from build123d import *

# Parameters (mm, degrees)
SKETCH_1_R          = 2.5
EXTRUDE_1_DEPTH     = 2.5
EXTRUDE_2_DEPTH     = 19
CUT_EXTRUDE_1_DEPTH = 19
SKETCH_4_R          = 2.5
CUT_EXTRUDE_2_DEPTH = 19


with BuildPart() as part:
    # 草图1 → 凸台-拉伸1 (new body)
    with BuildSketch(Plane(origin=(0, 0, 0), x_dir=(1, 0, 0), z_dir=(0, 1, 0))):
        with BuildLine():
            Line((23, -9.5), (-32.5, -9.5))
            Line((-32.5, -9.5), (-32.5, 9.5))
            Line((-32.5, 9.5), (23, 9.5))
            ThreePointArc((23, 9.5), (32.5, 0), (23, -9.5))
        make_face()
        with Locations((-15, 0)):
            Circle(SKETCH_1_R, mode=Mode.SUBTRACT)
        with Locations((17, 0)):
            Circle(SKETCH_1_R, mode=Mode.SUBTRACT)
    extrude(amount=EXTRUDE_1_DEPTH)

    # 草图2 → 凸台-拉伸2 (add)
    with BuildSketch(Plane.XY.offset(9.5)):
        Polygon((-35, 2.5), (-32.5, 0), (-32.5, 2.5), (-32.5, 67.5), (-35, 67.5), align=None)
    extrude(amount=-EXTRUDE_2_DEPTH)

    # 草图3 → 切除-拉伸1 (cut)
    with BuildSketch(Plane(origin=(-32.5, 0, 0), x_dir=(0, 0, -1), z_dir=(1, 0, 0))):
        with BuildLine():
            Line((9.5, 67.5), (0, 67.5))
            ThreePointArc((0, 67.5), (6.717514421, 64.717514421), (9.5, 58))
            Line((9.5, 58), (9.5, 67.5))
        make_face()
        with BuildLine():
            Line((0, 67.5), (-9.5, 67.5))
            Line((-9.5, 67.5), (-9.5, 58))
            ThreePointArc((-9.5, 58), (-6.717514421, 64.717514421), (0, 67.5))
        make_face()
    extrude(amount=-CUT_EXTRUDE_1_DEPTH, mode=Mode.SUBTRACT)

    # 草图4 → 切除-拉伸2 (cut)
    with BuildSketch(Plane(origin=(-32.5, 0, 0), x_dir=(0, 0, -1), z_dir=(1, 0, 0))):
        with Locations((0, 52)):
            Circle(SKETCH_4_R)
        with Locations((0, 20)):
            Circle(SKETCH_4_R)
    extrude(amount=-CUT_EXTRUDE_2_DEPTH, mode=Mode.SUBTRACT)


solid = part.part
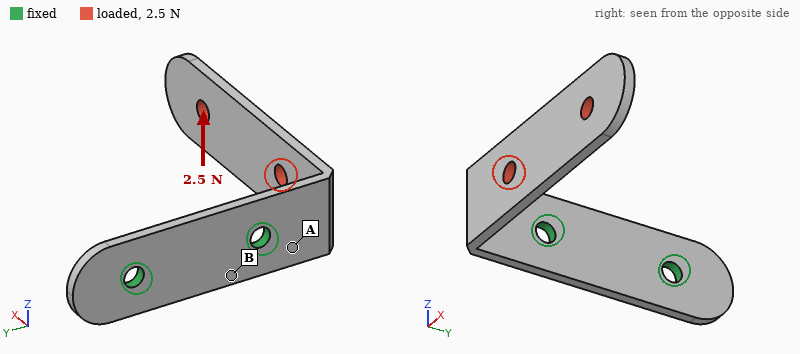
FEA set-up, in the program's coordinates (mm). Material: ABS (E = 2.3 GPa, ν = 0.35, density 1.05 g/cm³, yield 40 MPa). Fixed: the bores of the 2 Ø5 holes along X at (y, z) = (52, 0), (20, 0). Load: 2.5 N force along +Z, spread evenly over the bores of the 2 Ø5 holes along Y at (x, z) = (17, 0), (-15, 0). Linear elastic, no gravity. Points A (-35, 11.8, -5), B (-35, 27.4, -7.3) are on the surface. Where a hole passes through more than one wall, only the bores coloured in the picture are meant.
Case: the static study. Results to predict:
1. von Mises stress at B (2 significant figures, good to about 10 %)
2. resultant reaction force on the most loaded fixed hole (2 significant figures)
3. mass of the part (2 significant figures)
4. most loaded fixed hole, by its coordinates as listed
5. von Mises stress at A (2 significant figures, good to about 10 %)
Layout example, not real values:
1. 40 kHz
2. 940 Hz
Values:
1. 0.63 MPa
2. 3.4 N
3. 6.1 g
4. (20, 0)
5. 3.1 MPa
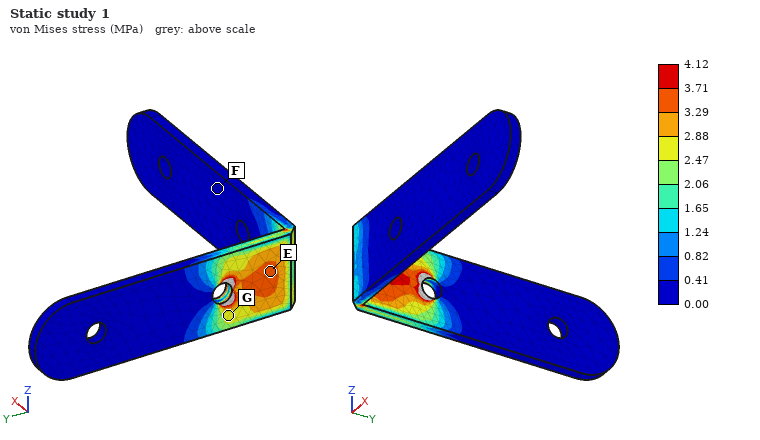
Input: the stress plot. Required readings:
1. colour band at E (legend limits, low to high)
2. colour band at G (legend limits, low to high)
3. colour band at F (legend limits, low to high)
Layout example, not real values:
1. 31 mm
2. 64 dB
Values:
1. 3.29 to 3.71 MPa
2. 2.47 to 2.88 MPa
3. 0.00 to 0.41 MPa
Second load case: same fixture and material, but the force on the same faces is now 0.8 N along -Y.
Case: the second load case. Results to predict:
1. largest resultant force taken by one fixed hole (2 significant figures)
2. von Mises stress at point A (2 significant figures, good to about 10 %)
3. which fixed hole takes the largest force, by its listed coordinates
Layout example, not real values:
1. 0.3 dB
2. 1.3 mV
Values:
1. 0.73 N
2. 1.3 MPa
3. (20, 0)
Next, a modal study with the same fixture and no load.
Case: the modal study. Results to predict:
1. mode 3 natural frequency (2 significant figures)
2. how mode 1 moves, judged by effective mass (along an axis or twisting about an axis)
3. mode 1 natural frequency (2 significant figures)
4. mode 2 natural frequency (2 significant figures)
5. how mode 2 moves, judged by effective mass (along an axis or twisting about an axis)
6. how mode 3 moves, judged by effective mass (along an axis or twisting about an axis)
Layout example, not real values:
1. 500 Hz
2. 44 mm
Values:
1. 550 Hz
2. along Y
3. 100 Hz
4. 170 Hz
5. along Z
6. along X
